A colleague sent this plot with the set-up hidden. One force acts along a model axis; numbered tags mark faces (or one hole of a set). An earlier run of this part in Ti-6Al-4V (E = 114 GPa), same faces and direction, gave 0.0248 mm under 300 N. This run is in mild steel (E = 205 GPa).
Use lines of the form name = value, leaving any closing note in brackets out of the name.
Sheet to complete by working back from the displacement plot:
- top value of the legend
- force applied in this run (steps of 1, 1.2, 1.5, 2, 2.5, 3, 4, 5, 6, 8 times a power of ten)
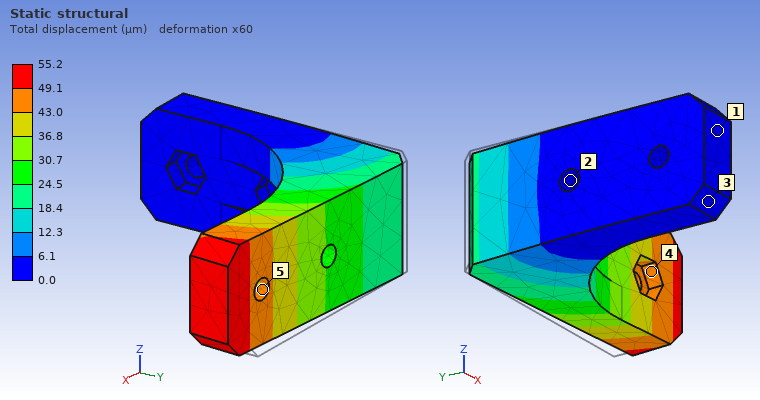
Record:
top value of the legend = 55.2 µm
force applied in this run = 1.2 kN
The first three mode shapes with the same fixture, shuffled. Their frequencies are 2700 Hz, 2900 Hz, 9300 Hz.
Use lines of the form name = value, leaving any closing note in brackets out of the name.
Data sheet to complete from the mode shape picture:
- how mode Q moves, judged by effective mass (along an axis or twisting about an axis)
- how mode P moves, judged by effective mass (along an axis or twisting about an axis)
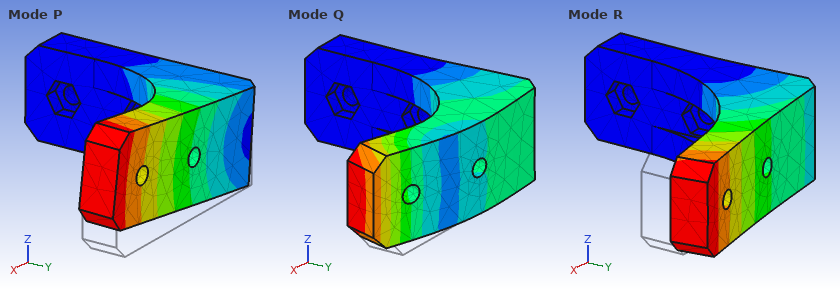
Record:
how mode Q moves, judged by effective mass = along X
how mode P moves, judged by effective mass = along Z
